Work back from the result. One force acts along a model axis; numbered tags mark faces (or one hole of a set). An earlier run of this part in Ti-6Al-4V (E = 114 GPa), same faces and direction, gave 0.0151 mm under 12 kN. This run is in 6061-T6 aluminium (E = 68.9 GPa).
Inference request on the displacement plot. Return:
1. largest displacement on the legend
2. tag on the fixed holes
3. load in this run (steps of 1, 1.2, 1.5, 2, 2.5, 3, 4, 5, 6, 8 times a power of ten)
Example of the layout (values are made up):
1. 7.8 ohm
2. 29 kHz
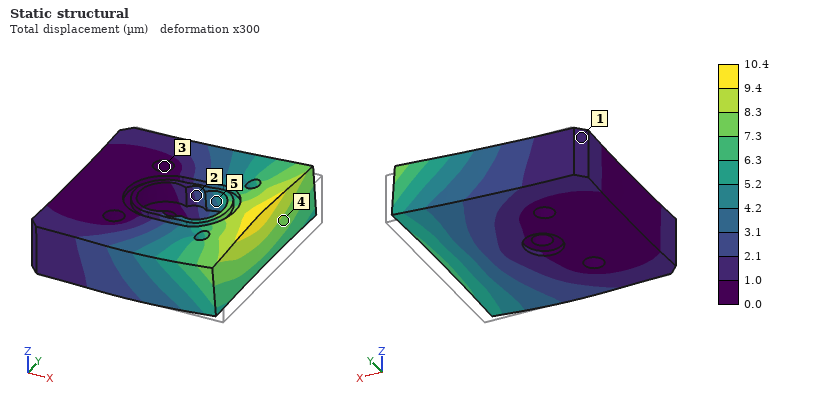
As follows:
1. 10.4 µm
2. 3
3. 5 kN
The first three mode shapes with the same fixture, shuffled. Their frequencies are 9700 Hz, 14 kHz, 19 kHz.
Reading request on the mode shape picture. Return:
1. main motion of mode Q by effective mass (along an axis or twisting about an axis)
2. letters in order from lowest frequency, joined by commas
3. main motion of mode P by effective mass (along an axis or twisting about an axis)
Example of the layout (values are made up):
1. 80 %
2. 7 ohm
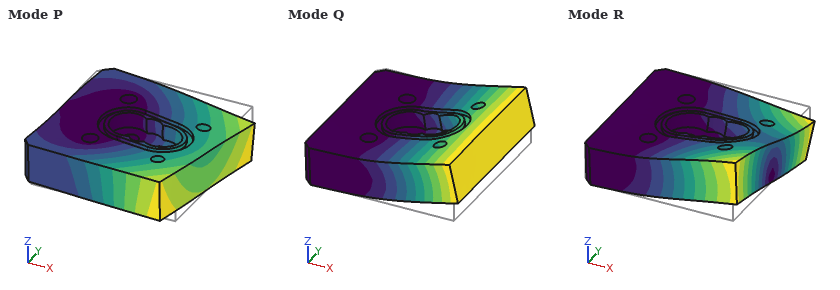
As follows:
1. along Z
2. Q, R, P
3. along Y
